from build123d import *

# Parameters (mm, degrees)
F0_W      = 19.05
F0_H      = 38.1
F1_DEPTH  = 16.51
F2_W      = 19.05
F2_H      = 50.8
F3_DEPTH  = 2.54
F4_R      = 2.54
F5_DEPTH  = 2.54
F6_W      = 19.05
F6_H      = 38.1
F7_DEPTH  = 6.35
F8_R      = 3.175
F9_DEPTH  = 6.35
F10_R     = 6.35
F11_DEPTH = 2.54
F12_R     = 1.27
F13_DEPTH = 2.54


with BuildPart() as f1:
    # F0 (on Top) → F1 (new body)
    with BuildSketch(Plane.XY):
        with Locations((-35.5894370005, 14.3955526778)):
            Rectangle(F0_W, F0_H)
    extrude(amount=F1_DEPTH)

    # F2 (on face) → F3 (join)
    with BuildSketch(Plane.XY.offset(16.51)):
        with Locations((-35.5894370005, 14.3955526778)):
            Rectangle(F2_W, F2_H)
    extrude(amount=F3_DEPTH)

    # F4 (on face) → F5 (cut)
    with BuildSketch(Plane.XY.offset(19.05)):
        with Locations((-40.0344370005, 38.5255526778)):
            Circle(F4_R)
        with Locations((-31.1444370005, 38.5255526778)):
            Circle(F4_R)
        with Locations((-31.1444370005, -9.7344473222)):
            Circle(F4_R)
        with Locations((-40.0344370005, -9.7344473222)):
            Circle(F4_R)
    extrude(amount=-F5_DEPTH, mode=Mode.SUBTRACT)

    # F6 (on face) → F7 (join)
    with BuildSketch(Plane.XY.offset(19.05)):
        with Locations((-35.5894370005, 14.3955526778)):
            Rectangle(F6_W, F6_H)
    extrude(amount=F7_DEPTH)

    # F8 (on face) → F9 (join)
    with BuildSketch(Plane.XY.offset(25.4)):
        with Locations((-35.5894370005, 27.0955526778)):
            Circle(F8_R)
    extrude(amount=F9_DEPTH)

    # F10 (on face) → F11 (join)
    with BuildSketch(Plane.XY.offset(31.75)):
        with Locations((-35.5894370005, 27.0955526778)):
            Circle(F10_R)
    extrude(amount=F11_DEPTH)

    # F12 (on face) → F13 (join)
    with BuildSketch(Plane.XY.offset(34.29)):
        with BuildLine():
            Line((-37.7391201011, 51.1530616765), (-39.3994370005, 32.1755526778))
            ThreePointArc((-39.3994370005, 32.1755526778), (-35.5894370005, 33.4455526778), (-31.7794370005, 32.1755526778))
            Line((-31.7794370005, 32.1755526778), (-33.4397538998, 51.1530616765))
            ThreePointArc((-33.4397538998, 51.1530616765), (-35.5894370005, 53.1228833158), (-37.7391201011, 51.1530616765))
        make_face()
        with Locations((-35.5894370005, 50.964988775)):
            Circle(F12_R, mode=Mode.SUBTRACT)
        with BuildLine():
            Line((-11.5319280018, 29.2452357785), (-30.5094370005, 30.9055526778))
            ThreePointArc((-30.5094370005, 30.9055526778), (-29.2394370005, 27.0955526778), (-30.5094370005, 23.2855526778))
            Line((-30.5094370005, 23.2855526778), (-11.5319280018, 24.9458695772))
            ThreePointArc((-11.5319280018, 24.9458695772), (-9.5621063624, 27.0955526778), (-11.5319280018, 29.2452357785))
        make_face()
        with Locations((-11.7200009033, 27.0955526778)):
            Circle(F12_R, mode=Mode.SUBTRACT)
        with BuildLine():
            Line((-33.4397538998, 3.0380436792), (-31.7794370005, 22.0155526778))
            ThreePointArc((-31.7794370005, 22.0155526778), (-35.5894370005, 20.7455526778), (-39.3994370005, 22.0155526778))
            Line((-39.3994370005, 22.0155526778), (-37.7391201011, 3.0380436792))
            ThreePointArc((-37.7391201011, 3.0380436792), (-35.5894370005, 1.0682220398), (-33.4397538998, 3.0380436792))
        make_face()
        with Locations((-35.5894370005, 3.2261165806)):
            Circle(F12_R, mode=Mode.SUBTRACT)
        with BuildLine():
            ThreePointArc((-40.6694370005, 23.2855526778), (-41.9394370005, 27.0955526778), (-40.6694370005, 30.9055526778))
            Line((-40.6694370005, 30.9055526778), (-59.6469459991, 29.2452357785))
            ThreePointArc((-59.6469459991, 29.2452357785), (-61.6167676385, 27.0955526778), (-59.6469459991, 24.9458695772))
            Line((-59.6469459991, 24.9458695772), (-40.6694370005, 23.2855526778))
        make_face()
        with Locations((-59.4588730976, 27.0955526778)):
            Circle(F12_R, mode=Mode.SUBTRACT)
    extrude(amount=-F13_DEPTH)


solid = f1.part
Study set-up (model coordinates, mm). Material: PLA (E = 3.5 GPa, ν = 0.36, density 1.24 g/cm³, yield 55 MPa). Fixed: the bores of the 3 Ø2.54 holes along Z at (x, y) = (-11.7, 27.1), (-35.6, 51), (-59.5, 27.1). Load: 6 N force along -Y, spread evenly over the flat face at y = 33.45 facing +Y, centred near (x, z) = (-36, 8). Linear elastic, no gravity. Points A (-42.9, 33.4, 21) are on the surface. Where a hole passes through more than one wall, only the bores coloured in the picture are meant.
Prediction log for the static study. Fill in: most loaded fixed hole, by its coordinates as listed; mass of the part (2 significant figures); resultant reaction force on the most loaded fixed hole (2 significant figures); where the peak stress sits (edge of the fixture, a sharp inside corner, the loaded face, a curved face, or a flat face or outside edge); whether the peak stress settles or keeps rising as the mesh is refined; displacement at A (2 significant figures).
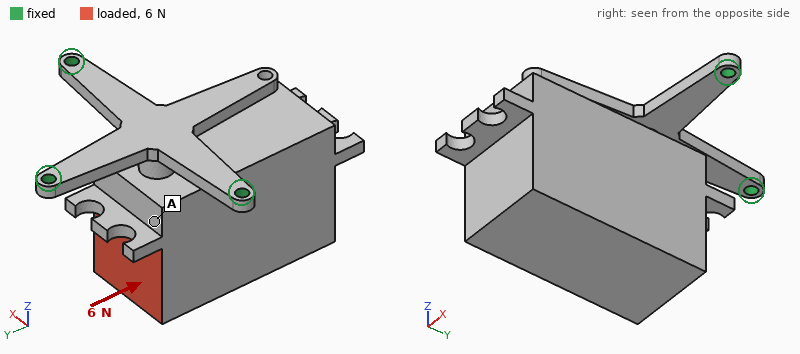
(-35.6, 51)
25 g
7.8 N
edge of the fixture
keeps rising
0.24 mm
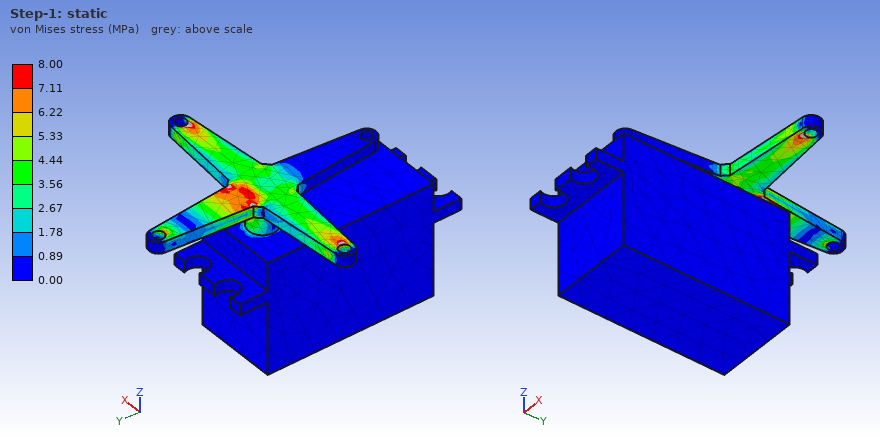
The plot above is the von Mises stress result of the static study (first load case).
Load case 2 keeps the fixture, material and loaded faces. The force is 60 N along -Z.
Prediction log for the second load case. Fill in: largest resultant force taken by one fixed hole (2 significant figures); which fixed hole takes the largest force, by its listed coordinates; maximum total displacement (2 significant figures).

24 N
(-35.6, 51)
0.90 mm
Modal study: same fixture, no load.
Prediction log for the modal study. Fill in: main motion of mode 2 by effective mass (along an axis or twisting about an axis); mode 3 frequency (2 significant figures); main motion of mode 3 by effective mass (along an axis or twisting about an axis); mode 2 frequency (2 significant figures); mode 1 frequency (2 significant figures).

along X
380 Hz
twisting about Z
160 Hz
94 Hz
